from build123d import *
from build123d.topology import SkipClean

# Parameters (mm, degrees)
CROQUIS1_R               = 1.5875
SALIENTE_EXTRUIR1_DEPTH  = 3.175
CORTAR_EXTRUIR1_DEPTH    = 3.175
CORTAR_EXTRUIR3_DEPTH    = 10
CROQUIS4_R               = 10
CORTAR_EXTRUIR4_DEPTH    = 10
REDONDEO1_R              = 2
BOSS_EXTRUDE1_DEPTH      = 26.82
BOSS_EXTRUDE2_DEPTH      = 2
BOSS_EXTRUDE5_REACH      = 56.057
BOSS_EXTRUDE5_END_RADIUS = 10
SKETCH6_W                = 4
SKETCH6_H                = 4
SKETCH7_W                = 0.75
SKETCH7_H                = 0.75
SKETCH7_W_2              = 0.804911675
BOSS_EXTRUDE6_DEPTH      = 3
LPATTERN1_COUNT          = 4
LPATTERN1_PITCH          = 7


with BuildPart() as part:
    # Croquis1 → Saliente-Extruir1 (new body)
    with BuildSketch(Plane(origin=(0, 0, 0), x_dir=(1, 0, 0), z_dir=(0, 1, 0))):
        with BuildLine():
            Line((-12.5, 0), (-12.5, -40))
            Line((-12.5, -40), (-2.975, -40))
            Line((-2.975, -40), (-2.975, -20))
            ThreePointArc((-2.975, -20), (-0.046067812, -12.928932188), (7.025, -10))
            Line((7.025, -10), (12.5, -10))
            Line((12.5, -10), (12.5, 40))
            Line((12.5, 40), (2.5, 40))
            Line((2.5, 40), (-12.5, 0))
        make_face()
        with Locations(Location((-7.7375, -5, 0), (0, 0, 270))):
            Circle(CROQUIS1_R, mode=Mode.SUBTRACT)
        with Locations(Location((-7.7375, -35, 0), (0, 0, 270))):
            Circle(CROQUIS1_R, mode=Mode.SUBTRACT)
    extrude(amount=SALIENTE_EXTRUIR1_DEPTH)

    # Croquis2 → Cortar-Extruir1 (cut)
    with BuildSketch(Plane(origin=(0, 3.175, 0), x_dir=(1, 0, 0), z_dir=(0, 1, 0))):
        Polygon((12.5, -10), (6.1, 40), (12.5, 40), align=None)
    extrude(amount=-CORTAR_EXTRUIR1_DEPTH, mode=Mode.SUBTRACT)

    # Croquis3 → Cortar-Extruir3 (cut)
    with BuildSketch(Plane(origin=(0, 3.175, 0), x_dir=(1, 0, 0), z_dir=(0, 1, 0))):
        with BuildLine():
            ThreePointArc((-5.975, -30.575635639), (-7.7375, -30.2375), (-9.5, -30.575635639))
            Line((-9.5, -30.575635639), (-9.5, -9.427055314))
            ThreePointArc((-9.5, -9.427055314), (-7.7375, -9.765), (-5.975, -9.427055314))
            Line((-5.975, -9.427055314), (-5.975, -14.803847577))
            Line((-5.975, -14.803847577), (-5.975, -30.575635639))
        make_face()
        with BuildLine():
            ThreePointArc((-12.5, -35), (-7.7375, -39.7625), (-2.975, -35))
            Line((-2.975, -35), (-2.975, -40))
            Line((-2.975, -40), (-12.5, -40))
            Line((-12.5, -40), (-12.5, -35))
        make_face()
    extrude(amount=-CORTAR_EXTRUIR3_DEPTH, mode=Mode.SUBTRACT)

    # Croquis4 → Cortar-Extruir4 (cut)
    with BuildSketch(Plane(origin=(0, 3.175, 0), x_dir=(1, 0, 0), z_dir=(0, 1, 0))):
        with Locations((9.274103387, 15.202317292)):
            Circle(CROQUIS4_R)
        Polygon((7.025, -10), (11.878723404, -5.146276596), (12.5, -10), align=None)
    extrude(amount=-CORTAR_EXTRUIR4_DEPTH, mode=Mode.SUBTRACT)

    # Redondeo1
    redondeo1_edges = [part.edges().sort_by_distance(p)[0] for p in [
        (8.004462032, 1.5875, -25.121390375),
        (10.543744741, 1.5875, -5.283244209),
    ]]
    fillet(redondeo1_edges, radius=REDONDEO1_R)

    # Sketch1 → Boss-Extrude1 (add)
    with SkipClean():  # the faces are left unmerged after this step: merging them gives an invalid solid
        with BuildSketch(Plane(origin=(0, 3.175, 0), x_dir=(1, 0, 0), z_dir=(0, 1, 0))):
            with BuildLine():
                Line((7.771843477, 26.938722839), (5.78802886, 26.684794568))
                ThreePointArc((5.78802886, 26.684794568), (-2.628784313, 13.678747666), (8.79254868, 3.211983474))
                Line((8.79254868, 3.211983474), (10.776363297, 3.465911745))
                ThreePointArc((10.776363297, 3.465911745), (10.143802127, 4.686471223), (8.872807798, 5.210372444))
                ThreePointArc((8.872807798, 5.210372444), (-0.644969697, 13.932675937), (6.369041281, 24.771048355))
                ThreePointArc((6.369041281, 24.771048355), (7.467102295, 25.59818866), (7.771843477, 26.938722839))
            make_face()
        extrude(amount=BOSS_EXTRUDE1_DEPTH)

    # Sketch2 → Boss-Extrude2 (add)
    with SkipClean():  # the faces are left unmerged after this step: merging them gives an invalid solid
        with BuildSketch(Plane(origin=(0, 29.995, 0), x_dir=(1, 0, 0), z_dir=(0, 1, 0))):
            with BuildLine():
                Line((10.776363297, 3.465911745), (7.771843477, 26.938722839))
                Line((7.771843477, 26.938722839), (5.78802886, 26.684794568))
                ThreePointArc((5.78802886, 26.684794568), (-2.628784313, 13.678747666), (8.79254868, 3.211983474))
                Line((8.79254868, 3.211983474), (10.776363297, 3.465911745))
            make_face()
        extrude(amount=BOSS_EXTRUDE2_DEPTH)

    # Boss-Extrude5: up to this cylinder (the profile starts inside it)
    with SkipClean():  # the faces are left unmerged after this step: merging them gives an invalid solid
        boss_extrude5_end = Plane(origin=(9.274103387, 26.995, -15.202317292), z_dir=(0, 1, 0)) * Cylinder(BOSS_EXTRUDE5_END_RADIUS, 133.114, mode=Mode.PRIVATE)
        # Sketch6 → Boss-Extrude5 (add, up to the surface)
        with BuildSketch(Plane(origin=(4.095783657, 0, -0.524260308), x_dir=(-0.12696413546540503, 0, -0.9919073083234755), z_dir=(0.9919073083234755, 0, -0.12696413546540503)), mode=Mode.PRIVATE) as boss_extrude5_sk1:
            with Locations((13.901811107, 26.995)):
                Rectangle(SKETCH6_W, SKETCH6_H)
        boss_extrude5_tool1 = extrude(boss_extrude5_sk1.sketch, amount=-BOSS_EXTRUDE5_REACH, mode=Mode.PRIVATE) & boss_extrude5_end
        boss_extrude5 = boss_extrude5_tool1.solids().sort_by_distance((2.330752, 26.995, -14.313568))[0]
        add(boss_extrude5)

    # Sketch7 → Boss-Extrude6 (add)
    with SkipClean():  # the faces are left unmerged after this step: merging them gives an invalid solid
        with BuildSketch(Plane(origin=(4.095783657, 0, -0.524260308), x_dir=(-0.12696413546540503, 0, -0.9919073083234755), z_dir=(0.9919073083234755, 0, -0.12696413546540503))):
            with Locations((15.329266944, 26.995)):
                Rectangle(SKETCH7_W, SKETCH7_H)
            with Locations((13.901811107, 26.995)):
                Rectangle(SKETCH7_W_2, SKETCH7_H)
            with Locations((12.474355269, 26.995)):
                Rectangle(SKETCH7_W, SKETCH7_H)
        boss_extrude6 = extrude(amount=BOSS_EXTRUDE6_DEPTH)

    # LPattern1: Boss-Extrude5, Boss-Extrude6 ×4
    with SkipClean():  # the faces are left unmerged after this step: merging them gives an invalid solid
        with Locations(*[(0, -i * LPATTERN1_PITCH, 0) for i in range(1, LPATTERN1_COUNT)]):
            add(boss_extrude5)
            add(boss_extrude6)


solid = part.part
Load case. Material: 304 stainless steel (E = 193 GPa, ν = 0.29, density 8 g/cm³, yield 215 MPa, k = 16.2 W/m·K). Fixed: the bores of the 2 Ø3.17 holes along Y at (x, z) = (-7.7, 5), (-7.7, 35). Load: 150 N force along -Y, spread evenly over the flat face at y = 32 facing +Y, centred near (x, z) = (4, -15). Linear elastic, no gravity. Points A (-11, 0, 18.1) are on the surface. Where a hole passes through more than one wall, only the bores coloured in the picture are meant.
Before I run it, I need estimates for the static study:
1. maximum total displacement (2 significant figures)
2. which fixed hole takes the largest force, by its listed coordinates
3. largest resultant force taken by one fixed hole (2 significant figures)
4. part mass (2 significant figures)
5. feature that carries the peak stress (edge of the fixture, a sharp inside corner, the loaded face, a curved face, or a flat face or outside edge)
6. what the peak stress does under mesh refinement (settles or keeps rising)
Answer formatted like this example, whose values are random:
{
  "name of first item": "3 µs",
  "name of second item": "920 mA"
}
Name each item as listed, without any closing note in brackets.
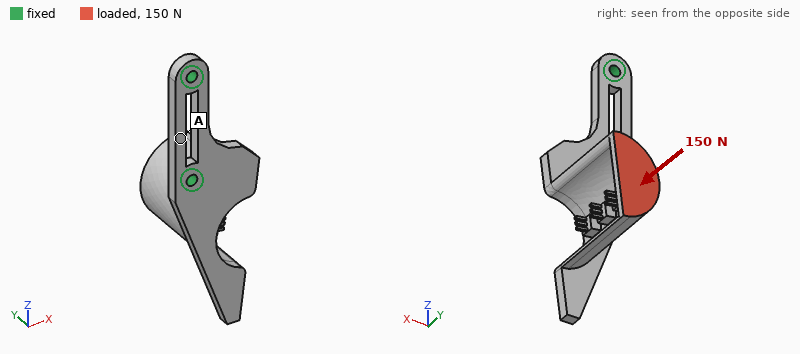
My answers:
{
  "maximum total displacement": "0.18 mm",
  "which fixed hole takes the largest force, by its listed coordinates": "(-7.7, 5)",
  "largest resultant force taken by one fixed hole": "170 N",
  "part mass": "41 g",
  "feature that carries the peak stress": "edge of the fixture",
  "what the peak stress does under mesh refinement": "keeps rising"
}
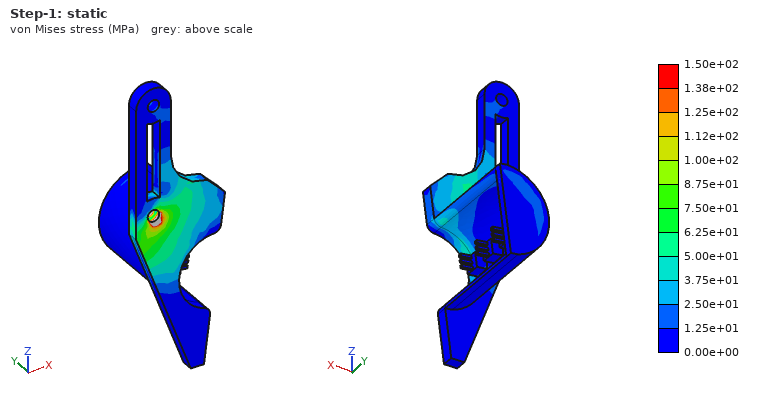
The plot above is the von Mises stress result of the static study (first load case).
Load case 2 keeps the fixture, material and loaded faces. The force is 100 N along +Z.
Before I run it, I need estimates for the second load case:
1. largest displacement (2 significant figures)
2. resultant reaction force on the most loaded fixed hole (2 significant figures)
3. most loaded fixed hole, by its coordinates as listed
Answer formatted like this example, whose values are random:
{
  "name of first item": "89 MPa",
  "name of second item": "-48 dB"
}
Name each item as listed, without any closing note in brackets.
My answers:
{
  "largest displacement": "0.23 mm",
  "resultant reaction force on the most loaded fixed hole": "77 N",
  "most loaded fixed hole, by its coordinates as listed": "(-7.7, 5)"
}
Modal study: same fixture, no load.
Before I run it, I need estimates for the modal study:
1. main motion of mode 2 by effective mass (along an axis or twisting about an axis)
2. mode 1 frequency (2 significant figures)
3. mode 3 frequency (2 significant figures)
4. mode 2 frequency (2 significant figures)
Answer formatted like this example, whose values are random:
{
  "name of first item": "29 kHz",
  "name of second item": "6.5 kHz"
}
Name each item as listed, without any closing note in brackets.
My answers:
{
  "main motion of mode 2 by effective mass": "along X",
  "mode 1 frequency": "900 Hz",
  "mode 3 frequency": "3200 Hz",
  "mode 2 frequency": "1400 Hz"
}
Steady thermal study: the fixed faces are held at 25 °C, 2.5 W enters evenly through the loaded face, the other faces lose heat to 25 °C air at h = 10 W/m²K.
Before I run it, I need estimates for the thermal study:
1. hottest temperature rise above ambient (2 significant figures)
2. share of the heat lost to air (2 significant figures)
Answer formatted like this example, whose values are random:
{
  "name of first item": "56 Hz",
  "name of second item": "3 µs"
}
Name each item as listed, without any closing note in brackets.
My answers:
{
  "hottest temperature rise above ambient": "77 K",
  "share of the heat lost to air": "57 %"
}
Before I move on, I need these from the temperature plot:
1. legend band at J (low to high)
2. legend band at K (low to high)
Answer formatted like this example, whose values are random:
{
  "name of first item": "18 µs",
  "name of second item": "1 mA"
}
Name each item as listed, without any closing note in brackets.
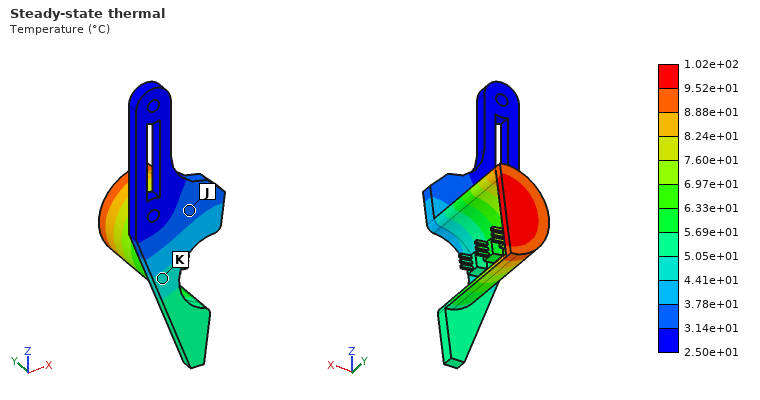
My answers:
{
  "legend band at J": "3.14e+01 to 3.78e+01 °C",
  "legend band at K": "4.41e+01 to 5.05e+01 °C"
}
